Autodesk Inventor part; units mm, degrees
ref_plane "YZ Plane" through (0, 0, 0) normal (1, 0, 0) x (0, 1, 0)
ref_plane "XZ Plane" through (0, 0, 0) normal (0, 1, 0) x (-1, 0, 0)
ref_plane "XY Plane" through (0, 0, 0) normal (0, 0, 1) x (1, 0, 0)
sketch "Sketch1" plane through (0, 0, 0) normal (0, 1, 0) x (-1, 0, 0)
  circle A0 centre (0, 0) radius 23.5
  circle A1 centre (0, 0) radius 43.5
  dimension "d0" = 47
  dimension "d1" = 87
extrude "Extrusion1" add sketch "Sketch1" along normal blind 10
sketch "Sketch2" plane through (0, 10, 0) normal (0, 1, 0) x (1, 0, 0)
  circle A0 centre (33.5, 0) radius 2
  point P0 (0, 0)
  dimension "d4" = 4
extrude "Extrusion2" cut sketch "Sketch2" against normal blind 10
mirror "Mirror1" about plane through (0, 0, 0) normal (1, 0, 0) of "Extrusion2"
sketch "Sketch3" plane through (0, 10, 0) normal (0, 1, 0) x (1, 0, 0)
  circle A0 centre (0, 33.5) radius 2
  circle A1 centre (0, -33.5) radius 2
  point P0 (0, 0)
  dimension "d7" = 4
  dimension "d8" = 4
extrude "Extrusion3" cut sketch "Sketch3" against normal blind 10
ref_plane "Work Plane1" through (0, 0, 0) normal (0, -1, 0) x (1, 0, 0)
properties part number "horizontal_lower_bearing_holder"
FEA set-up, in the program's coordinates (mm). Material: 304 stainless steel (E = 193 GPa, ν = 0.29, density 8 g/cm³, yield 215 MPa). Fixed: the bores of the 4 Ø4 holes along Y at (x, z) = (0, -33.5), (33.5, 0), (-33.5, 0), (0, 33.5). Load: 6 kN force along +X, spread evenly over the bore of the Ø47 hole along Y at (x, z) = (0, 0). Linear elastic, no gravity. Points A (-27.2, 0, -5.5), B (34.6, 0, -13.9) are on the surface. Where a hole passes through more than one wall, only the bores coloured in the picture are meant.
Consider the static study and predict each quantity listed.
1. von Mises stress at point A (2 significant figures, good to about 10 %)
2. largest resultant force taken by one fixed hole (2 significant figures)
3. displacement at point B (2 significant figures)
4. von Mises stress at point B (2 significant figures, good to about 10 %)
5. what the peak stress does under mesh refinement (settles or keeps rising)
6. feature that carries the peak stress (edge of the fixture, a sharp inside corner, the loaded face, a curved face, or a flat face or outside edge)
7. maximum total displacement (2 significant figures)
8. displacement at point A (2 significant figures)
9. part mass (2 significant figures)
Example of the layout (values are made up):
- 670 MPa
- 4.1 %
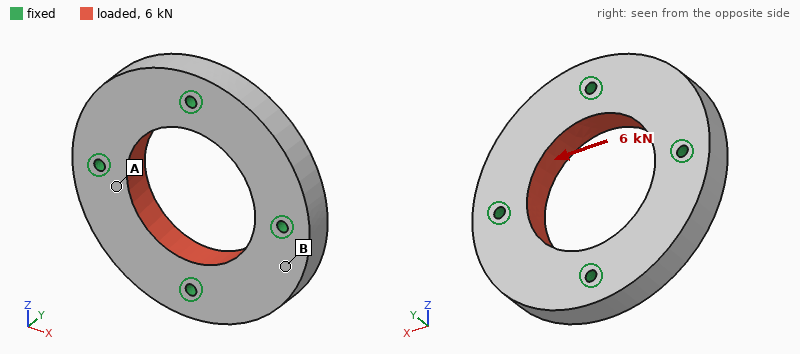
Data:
- 8.0 MPa
- 1.7 kN
- 0.64 µm
- 3.4 MPa
- keeps rising
- edge of the fixture
- 1.1 µm
- 0.44 µm
- 330 g
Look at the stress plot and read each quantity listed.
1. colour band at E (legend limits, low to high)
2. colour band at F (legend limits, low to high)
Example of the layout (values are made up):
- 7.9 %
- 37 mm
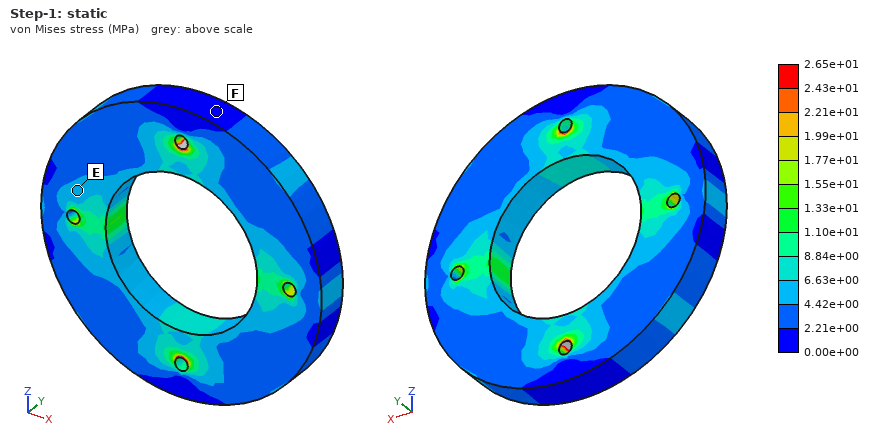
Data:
- 4.42e+00 to 6.63e+00 MPa
- 0.00e+00 to 2.21e+00 MPa
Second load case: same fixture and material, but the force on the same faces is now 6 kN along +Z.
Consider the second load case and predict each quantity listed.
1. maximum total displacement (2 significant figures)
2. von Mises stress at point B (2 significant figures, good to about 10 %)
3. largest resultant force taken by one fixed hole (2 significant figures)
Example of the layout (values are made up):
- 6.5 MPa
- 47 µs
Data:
- 1.1 µm
- 4.1 MPa
- 1.7 kN
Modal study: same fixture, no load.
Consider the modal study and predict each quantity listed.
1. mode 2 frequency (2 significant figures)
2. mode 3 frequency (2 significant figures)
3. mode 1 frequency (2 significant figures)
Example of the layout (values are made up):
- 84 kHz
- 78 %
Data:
- 12 kHz
- 12 kHz
- 11 kHz
